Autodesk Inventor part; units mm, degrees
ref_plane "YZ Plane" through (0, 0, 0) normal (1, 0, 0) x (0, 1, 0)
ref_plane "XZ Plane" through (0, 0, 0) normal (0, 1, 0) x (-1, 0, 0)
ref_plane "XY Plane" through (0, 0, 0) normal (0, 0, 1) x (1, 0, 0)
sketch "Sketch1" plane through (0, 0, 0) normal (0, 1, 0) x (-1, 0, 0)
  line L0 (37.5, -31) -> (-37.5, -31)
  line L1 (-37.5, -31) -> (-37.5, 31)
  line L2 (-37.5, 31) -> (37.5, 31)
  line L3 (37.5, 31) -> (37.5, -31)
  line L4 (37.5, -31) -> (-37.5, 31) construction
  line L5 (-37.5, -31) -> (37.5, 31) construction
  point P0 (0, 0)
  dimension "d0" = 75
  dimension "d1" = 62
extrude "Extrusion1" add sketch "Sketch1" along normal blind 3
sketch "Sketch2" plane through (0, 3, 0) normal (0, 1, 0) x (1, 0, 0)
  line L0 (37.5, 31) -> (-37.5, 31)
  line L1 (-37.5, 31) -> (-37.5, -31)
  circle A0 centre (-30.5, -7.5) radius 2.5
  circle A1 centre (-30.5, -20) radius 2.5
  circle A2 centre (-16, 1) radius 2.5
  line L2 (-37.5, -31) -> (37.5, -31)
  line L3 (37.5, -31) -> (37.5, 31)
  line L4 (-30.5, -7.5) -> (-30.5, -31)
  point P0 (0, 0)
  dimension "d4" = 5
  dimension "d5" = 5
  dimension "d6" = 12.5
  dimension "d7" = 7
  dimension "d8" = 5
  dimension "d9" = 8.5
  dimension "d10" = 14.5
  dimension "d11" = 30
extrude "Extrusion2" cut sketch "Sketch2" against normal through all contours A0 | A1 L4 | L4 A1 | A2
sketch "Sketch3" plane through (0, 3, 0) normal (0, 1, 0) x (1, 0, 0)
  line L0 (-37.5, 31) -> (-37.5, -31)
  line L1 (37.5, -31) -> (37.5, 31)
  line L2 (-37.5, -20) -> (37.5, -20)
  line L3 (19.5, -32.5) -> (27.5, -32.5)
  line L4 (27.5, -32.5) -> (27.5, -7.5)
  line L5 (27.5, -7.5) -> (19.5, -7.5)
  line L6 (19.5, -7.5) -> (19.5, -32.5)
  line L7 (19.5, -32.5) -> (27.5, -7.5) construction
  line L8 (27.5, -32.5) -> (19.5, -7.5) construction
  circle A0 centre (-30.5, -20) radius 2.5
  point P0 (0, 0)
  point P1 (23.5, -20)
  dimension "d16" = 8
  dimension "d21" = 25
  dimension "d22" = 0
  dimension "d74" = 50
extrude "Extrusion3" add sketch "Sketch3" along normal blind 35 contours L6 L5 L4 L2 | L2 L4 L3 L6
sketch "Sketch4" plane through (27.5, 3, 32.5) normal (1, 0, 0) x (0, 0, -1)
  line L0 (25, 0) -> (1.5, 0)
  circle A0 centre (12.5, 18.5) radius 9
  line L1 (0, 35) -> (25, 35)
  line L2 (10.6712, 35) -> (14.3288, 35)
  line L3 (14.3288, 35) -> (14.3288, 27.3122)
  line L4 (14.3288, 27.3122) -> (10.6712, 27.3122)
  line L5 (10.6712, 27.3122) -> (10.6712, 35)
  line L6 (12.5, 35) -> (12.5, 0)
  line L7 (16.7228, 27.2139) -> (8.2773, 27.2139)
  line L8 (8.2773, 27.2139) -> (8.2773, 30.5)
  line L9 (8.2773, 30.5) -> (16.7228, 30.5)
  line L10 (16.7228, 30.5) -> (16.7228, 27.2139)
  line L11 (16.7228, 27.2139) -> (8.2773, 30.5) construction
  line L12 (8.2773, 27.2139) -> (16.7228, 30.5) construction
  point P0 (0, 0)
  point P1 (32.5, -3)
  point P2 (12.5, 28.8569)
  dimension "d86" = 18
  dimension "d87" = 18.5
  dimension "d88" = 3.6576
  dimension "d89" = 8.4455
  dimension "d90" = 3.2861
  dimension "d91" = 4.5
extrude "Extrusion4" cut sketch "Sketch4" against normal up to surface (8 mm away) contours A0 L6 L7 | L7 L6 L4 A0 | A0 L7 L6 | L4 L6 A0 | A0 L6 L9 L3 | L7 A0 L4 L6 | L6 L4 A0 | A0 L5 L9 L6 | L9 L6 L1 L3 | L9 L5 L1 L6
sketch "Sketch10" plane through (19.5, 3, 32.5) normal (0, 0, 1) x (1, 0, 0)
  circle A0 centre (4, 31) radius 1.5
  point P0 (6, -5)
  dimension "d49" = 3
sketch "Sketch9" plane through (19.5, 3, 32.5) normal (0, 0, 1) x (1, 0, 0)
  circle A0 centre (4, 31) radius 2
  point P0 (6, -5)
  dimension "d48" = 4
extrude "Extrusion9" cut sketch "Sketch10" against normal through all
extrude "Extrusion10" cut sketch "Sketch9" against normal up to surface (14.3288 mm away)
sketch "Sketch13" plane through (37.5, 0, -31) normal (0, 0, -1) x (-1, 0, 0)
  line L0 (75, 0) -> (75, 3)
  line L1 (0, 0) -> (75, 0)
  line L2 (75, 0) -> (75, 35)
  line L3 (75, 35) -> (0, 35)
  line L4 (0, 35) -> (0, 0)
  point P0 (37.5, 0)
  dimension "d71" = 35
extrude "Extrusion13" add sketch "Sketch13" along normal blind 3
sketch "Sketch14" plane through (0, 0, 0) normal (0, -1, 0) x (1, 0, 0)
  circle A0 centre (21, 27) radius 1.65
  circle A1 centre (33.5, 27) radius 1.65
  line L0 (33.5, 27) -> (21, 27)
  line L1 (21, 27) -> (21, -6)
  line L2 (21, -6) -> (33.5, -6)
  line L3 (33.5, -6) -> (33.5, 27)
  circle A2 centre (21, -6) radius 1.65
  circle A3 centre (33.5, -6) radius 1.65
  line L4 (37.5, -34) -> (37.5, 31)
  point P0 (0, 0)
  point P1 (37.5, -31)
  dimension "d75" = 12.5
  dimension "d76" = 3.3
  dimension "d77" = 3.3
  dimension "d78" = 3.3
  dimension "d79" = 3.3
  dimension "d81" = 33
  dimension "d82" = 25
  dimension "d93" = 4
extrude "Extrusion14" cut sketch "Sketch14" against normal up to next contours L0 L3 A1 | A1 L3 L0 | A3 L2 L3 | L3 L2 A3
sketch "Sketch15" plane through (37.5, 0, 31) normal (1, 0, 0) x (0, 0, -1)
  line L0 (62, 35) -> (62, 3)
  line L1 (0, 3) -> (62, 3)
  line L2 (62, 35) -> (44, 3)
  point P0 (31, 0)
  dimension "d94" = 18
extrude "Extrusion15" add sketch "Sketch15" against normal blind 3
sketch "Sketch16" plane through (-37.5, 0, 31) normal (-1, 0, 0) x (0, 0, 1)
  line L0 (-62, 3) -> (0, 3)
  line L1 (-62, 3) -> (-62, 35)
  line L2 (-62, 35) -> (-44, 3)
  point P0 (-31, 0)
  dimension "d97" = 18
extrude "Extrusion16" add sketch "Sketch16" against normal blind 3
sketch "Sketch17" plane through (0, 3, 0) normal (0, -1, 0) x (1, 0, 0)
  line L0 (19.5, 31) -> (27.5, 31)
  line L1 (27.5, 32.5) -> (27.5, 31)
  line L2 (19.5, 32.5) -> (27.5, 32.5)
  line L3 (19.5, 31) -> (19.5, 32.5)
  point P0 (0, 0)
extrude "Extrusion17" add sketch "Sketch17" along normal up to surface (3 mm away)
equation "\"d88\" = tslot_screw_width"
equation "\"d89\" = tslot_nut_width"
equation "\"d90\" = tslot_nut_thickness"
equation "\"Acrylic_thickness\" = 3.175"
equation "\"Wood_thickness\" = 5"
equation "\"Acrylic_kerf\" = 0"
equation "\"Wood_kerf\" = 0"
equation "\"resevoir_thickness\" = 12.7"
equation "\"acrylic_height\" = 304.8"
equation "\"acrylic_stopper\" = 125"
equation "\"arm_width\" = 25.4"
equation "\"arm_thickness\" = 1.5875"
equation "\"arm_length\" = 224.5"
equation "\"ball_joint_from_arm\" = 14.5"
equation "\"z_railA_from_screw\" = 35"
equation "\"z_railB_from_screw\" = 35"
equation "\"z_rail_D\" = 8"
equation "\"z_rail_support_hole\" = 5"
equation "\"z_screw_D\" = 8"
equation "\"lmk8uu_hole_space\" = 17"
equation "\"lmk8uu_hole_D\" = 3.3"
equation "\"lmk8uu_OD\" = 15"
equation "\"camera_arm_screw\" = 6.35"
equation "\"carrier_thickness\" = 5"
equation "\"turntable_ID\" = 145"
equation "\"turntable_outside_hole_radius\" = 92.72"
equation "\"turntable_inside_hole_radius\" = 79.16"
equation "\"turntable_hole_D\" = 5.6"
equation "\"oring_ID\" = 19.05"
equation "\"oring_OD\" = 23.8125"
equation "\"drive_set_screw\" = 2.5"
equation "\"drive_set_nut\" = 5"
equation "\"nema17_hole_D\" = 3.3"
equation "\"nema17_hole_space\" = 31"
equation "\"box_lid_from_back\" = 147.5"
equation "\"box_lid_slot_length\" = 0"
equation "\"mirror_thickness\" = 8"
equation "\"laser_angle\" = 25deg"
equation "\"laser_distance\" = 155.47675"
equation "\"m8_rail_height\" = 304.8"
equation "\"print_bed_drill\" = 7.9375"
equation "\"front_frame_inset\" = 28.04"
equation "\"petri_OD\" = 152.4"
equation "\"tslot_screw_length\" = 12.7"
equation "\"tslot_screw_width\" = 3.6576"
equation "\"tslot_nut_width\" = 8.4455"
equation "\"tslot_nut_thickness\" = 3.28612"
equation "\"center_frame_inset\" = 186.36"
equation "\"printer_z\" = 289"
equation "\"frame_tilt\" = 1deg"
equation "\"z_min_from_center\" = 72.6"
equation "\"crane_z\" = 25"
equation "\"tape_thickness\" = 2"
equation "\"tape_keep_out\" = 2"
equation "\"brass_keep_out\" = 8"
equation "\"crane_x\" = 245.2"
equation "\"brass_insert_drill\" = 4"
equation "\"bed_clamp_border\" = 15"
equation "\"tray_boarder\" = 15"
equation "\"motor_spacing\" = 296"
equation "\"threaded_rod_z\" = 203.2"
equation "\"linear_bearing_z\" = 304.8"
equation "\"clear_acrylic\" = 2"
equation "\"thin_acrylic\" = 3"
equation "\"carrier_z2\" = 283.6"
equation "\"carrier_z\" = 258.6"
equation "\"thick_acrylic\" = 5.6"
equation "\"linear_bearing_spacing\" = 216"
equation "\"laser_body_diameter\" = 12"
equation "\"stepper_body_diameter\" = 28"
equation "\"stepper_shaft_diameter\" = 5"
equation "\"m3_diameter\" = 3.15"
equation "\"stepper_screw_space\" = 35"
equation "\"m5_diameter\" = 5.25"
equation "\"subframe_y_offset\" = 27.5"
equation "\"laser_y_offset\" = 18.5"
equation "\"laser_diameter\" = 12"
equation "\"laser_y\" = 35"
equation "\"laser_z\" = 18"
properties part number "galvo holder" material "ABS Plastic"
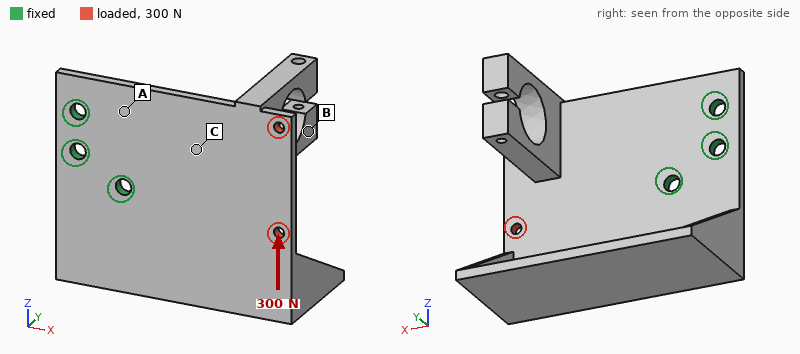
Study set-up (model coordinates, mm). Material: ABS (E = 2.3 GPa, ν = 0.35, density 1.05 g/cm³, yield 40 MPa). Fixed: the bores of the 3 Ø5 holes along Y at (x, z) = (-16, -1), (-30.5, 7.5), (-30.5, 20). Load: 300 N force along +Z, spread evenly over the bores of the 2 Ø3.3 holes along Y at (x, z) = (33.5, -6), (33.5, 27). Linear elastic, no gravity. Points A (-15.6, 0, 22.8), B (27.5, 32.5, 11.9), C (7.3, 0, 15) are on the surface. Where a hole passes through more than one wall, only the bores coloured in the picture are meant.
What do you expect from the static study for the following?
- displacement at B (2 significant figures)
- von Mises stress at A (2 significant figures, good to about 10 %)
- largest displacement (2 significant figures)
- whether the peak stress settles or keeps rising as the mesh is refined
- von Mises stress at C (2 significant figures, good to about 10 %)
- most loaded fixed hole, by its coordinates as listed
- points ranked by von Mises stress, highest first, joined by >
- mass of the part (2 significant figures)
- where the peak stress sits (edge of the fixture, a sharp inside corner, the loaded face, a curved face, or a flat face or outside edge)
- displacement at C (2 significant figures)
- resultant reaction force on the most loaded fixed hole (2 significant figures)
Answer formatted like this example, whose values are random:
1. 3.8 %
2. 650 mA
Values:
1. 0.40 mm
2. 7.9 MPa
3. 0.60 mm
4. keeps rising
5. 4.4 MPa
6. (-16, -1)
7. A > C > B
8. 29 g
9. edge of the fixture
10. 0.23 mm
11. 710 N
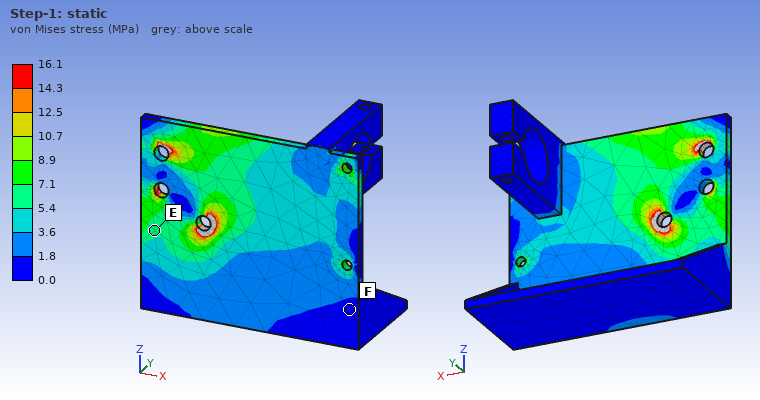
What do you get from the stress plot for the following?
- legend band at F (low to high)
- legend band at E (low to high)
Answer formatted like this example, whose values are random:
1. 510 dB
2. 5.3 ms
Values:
1. 0.0 to 1.8 MPa
2. 5.4 to 7.1 MPa
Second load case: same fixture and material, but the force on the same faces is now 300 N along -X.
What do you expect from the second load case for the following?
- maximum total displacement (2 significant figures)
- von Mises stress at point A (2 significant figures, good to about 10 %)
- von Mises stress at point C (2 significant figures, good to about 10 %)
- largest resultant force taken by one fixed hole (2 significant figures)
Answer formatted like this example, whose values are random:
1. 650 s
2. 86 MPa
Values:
1. 0.13 mm
2. 2.6 MPa
3. 2.1 MPa
4. 130 N
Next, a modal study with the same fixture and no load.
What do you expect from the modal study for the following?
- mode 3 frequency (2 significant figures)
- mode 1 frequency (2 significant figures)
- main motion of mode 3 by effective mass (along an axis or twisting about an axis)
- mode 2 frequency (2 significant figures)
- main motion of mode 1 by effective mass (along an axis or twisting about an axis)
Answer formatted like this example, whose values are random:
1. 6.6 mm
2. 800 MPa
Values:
1. 300 Hz
2. 150 Hz
3. along Y
4. 170 Hz
5. along Y
